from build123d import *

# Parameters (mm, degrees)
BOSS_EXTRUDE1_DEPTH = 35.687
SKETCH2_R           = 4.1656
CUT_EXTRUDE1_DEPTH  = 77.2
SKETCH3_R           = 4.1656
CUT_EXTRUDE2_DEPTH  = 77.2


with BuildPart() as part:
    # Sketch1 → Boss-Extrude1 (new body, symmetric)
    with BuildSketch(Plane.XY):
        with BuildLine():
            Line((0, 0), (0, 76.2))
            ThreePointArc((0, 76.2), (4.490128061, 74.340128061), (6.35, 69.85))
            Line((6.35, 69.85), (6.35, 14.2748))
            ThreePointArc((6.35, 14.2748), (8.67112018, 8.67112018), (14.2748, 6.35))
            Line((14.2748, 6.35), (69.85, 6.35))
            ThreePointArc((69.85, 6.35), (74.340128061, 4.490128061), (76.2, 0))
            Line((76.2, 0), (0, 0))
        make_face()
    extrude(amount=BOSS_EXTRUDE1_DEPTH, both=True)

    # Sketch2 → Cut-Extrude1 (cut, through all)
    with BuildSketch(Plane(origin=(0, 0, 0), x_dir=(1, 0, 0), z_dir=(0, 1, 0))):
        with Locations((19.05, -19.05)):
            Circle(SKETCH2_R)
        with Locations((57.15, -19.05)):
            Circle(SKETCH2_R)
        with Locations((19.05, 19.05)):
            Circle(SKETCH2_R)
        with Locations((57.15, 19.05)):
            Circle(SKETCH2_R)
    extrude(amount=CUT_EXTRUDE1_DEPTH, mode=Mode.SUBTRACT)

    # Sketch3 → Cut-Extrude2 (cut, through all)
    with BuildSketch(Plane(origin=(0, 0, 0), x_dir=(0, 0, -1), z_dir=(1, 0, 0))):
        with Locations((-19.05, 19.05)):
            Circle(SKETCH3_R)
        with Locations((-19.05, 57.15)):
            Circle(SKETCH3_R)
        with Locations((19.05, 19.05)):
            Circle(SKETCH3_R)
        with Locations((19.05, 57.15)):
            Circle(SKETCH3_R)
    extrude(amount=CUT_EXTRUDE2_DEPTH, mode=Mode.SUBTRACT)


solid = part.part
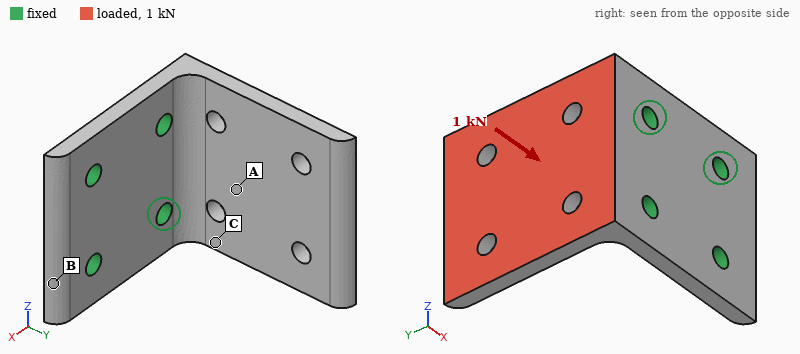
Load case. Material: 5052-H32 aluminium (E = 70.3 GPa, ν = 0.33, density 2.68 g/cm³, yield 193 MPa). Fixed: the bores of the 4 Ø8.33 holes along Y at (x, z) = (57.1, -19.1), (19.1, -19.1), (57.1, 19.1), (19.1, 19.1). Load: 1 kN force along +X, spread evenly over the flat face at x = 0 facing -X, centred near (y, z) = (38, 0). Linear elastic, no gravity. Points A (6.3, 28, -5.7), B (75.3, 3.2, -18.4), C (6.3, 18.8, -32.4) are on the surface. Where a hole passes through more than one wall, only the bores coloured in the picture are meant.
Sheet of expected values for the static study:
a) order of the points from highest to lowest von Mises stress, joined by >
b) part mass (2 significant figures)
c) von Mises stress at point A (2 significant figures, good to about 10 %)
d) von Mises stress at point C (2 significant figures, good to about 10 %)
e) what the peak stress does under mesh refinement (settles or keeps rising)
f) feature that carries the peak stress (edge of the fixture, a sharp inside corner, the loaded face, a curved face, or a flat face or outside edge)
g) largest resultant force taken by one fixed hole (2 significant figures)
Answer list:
C > A > B
170 g
32 MPa
51 MPa
keeps rising
edge of the fixture
460 N
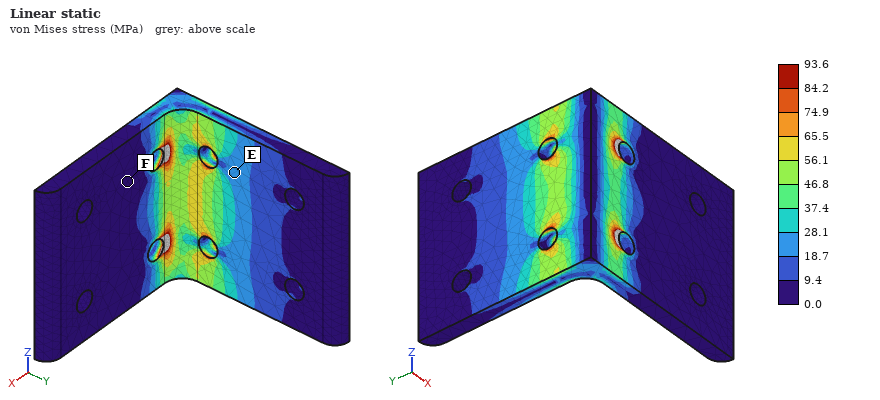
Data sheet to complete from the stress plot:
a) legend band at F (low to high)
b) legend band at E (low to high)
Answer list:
0.0 to 9.4 MPa
18.7 to 28.1 MPa
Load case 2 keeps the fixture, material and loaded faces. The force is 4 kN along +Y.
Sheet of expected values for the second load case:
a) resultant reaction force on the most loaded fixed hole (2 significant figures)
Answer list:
2.2 kN
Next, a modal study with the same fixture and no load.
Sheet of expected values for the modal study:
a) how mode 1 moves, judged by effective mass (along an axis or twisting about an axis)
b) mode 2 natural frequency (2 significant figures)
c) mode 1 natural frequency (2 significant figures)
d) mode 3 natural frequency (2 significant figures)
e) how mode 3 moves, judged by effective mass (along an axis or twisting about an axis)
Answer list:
along X
2200 Hz
900 Hz
3300 Hz
along Z
